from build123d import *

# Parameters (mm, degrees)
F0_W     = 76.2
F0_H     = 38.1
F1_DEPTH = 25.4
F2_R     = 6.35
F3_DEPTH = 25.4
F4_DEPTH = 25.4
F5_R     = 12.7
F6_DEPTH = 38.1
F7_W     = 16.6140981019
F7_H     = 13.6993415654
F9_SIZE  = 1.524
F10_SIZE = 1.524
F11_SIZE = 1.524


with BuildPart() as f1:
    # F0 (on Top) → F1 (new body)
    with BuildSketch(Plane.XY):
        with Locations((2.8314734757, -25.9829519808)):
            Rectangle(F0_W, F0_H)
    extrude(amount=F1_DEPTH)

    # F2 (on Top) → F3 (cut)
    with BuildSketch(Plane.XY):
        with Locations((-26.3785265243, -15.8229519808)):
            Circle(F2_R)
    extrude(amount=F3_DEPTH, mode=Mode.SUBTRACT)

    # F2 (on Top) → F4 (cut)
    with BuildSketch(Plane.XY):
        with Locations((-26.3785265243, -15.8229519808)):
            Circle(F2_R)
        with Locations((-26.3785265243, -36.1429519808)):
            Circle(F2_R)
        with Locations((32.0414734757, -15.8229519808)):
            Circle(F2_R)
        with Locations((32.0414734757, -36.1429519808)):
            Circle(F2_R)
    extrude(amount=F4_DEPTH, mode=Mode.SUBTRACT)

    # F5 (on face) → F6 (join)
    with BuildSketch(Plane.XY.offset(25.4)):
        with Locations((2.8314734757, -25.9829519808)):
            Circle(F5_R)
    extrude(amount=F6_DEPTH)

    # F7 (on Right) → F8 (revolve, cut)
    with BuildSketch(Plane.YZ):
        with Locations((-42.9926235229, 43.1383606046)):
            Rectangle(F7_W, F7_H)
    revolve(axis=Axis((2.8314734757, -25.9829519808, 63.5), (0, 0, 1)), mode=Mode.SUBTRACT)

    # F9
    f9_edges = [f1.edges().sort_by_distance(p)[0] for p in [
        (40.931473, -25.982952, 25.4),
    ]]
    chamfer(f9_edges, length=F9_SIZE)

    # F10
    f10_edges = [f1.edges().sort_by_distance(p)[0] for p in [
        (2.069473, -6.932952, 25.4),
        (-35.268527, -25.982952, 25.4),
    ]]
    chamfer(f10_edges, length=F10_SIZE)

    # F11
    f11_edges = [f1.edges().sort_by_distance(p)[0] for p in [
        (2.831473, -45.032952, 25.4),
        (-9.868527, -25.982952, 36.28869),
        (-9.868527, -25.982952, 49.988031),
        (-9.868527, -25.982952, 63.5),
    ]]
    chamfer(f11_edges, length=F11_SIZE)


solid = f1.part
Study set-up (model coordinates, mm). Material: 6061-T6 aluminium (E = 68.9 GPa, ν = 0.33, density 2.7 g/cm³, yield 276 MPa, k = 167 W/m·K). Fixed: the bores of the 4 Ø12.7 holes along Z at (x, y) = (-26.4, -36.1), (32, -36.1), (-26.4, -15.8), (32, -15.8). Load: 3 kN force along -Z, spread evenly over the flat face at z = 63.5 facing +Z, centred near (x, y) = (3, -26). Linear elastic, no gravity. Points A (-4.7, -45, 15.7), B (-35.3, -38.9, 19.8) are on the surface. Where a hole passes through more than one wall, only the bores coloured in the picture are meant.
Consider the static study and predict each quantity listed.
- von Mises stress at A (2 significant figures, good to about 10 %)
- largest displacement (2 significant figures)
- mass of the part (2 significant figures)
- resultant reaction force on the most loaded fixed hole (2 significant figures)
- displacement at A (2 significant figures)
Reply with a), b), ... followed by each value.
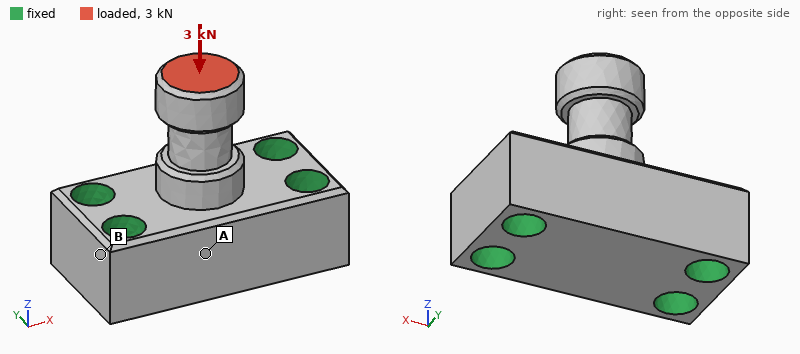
a) 2.3 MPa
b) 6.7 µm
c) 210 g
d) 780 N
e) 1.2 µm
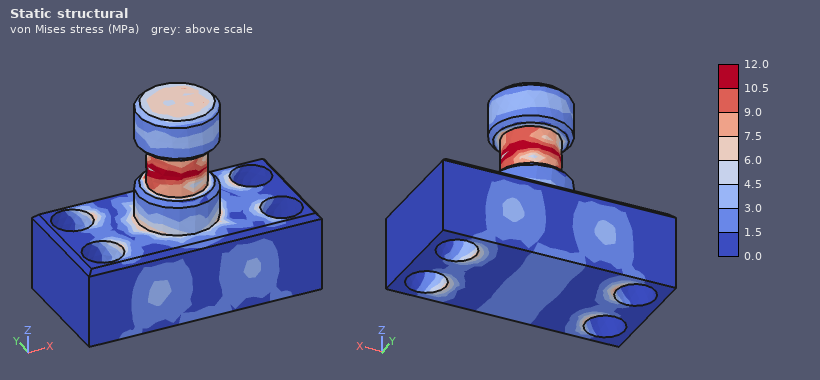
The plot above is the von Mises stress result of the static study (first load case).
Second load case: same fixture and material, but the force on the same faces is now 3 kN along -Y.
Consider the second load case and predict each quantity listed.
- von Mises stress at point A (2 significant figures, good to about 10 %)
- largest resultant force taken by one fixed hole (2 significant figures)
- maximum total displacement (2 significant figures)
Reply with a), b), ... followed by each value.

a) 17 MPa
b) 2.5 kN
c) 0.14 mm
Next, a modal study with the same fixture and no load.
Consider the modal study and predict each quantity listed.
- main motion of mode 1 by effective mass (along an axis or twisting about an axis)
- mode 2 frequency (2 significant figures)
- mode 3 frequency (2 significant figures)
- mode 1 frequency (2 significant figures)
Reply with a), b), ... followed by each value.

a) along Y
b) 7100 Hz
c) 15 kHz
d) 6500 Hz
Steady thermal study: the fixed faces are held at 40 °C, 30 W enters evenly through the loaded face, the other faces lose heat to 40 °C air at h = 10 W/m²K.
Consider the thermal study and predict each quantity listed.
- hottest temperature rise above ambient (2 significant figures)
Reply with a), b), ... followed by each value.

a) 23 K
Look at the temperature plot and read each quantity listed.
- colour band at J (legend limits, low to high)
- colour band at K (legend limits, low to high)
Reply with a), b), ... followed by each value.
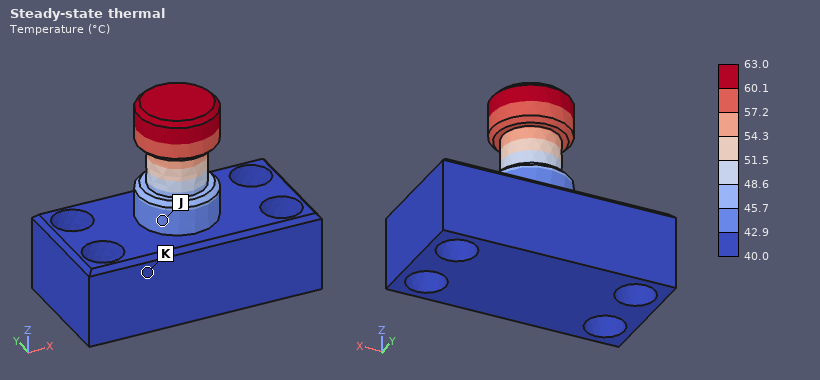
a) 42.9 to 45.7 °C
b) 40.0 to 42.9 °C
